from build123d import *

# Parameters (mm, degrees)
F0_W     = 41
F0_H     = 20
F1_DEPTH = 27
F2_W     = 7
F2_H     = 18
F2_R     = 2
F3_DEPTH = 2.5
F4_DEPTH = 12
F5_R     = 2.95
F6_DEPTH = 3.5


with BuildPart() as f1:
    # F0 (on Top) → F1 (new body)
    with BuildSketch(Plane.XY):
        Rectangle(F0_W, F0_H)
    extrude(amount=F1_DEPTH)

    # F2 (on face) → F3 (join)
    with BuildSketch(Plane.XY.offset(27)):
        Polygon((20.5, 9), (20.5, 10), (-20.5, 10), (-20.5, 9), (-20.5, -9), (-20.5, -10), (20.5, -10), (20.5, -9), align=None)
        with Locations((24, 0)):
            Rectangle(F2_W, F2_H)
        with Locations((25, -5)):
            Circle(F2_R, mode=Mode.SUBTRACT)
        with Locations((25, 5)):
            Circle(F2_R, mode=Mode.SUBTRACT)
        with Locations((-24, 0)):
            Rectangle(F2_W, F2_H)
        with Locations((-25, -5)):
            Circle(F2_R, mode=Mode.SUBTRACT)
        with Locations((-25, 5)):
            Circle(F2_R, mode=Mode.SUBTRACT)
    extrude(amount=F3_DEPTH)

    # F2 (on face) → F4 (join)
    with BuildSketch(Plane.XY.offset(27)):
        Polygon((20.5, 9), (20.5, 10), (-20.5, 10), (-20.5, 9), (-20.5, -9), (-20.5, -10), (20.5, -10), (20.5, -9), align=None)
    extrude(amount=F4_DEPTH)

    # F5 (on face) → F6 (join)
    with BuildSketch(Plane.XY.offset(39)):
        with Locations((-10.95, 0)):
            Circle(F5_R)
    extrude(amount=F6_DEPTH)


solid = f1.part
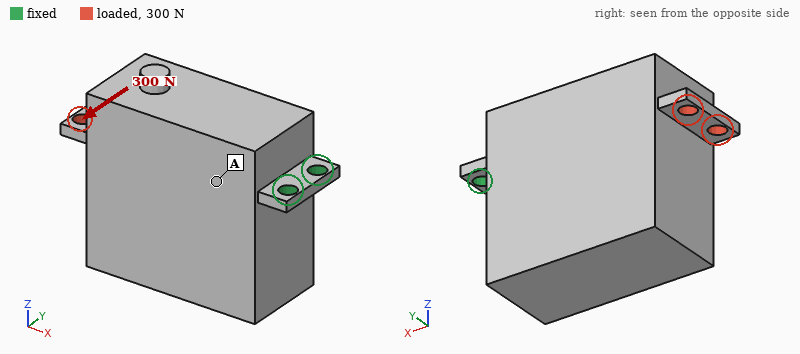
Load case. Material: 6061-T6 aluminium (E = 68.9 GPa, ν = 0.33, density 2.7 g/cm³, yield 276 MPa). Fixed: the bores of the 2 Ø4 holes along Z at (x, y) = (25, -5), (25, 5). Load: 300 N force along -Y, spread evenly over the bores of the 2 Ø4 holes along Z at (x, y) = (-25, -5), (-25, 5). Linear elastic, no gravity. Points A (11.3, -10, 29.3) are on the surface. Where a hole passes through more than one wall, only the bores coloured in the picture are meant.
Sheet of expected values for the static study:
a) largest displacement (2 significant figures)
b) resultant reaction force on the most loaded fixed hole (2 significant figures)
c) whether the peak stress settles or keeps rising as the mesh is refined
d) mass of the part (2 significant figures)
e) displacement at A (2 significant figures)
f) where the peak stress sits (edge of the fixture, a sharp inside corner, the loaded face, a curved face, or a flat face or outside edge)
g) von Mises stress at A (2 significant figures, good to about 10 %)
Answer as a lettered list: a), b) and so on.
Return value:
a) 65 µm
b) 1.2 kN
c) keeps rising
d) 88 g
e) 17 µm
f) edge of the fixture
g) 11 MPa
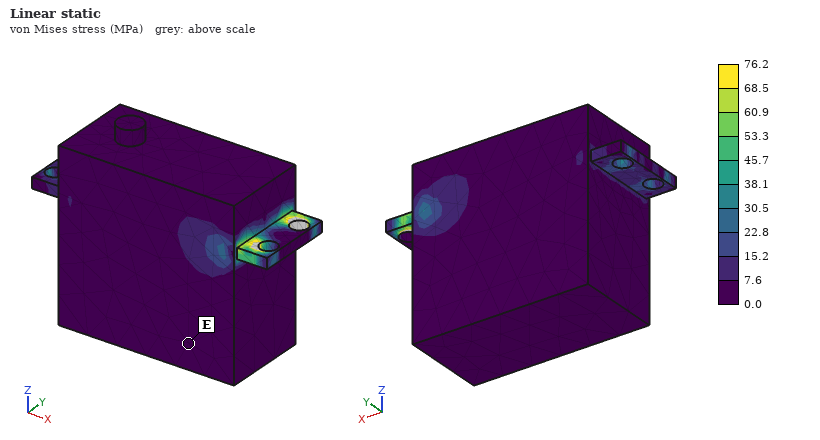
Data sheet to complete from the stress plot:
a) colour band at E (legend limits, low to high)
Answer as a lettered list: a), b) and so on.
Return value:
a) 0.0 to 7.6 MPa
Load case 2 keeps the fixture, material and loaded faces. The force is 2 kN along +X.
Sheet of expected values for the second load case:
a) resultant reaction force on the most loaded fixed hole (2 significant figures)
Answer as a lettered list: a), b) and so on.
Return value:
a) 1.0 kN
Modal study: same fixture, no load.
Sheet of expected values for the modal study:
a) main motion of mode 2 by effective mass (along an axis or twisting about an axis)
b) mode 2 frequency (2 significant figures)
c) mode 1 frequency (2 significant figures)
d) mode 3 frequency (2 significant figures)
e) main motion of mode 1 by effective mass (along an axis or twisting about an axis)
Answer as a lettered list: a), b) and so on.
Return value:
a) along Y
b) 1900 Hz
c) 390 Hz
d) 3100 Hz
e) along Z
